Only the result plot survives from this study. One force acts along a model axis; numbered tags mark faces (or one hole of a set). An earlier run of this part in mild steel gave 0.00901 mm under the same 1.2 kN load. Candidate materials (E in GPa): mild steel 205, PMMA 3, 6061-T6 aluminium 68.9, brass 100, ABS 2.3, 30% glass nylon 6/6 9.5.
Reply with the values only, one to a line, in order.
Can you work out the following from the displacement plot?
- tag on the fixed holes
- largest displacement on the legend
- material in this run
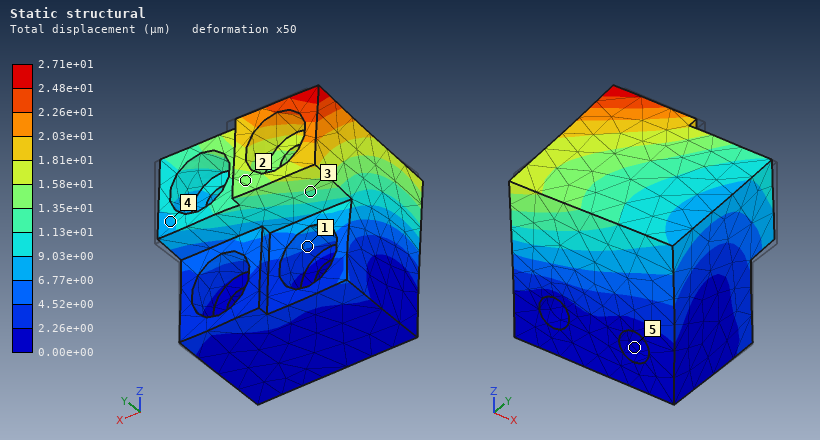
5
2.71e+01 µm
6061-T6 aluminium
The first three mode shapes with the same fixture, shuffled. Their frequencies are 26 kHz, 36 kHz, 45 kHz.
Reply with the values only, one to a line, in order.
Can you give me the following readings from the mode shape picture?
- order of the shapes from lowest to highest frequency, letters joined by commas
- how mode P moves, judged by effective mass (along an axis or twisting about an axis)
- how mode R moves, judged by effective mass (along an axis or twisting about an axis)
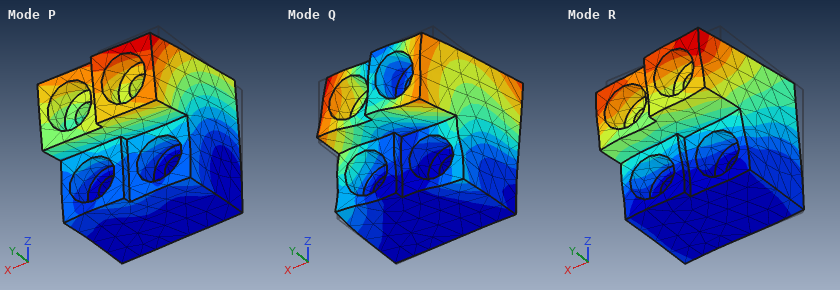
P, R, Q
along Y
along X
